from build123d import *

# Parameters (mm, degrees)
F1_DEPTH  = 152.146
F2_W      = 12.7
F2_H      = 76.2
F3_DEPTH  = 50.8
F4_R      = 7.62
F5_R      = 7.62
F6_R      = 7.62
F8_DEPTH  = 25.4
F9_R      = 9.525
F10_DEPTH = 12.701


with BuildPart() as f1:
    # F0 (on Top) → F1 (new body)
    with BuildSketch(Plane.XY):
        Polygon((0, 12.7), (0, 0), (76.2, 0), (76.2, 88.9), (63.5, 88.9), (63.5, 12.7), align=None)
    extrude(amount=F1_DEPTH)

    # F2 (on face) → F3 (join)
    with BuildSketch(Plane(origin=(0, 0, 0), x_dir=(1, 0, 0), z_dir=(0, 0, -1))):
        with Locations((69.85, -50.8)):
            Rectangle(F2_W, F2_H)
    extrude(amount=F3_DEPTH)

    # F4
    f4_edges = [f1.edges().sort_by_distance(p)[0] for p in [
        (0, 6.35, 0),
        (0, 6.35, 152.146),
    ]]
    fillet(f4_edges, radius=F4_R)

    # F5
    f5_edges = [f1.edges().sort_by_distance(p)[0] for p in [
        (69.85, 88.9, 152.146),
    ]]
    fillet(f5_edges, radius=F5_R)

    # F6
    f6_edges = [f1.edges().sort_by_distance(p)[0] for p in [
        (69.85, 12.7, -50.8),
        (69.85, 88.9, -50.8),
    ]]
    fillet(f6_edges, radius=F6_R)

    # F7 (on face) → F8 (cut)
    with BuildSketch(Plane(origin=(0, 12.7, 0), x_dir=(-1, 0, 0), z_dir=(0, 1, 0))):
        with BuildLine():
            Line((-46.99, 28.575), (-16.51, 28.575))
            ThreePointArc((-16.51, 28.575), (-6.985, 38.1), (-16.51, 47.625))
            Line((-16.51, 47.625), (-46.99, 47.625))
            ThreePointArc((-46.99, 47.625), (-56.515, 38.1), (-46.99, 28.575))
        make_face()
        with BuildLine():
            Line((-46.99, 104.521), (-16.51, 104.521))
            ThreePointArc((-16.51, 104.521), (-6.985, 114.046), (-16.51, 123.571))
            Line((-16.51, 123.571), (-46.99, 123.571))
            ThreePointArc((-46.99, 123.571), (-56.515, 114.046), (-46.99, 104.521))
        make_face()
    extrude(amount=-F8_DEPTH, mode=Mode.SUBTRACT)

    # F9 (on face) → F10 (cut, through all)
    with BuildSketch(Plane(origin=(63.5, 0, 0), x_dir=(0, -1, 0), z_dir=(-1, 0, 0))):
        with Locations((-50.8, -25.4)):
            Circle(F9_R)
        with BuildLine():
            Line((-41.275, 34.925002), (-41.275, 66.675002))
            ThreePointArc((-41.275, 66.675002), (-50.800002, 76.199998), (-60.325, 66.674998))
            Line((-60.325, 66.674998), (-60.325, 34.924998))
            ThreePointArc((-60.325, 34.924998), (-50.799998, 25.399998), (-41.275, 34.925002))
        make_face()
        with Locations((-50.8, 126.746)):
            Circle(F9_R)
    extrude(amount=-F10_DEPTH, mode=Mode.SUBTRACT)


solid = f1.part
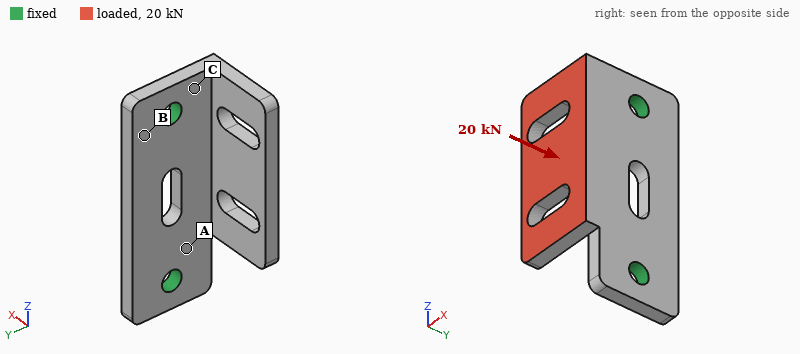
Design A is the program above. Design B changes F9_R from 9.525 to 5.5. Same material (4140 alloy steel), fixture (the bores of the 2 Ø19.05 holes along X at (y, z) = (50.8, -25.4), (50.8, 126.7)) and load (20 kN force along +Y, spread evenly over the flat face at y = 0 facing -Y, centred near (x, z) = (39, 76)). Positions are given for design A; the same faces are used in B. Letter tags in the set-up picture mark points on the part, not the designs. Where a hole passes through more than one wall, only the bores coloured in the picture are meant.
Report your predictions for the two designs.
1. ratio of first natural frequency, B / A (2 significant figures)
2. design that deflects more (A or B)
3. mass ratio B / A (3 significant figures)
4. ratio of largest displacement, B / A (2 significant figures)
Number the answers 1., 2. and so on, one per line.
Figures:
1. 0.91
2. B
3. 1.02
4. 1.1
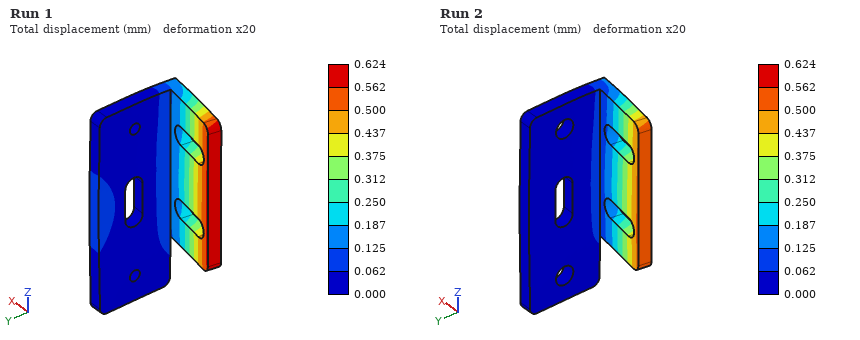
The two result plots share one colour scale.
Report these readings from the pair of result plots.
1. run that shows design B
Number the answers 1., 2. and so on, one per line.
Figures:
1. Run 1
